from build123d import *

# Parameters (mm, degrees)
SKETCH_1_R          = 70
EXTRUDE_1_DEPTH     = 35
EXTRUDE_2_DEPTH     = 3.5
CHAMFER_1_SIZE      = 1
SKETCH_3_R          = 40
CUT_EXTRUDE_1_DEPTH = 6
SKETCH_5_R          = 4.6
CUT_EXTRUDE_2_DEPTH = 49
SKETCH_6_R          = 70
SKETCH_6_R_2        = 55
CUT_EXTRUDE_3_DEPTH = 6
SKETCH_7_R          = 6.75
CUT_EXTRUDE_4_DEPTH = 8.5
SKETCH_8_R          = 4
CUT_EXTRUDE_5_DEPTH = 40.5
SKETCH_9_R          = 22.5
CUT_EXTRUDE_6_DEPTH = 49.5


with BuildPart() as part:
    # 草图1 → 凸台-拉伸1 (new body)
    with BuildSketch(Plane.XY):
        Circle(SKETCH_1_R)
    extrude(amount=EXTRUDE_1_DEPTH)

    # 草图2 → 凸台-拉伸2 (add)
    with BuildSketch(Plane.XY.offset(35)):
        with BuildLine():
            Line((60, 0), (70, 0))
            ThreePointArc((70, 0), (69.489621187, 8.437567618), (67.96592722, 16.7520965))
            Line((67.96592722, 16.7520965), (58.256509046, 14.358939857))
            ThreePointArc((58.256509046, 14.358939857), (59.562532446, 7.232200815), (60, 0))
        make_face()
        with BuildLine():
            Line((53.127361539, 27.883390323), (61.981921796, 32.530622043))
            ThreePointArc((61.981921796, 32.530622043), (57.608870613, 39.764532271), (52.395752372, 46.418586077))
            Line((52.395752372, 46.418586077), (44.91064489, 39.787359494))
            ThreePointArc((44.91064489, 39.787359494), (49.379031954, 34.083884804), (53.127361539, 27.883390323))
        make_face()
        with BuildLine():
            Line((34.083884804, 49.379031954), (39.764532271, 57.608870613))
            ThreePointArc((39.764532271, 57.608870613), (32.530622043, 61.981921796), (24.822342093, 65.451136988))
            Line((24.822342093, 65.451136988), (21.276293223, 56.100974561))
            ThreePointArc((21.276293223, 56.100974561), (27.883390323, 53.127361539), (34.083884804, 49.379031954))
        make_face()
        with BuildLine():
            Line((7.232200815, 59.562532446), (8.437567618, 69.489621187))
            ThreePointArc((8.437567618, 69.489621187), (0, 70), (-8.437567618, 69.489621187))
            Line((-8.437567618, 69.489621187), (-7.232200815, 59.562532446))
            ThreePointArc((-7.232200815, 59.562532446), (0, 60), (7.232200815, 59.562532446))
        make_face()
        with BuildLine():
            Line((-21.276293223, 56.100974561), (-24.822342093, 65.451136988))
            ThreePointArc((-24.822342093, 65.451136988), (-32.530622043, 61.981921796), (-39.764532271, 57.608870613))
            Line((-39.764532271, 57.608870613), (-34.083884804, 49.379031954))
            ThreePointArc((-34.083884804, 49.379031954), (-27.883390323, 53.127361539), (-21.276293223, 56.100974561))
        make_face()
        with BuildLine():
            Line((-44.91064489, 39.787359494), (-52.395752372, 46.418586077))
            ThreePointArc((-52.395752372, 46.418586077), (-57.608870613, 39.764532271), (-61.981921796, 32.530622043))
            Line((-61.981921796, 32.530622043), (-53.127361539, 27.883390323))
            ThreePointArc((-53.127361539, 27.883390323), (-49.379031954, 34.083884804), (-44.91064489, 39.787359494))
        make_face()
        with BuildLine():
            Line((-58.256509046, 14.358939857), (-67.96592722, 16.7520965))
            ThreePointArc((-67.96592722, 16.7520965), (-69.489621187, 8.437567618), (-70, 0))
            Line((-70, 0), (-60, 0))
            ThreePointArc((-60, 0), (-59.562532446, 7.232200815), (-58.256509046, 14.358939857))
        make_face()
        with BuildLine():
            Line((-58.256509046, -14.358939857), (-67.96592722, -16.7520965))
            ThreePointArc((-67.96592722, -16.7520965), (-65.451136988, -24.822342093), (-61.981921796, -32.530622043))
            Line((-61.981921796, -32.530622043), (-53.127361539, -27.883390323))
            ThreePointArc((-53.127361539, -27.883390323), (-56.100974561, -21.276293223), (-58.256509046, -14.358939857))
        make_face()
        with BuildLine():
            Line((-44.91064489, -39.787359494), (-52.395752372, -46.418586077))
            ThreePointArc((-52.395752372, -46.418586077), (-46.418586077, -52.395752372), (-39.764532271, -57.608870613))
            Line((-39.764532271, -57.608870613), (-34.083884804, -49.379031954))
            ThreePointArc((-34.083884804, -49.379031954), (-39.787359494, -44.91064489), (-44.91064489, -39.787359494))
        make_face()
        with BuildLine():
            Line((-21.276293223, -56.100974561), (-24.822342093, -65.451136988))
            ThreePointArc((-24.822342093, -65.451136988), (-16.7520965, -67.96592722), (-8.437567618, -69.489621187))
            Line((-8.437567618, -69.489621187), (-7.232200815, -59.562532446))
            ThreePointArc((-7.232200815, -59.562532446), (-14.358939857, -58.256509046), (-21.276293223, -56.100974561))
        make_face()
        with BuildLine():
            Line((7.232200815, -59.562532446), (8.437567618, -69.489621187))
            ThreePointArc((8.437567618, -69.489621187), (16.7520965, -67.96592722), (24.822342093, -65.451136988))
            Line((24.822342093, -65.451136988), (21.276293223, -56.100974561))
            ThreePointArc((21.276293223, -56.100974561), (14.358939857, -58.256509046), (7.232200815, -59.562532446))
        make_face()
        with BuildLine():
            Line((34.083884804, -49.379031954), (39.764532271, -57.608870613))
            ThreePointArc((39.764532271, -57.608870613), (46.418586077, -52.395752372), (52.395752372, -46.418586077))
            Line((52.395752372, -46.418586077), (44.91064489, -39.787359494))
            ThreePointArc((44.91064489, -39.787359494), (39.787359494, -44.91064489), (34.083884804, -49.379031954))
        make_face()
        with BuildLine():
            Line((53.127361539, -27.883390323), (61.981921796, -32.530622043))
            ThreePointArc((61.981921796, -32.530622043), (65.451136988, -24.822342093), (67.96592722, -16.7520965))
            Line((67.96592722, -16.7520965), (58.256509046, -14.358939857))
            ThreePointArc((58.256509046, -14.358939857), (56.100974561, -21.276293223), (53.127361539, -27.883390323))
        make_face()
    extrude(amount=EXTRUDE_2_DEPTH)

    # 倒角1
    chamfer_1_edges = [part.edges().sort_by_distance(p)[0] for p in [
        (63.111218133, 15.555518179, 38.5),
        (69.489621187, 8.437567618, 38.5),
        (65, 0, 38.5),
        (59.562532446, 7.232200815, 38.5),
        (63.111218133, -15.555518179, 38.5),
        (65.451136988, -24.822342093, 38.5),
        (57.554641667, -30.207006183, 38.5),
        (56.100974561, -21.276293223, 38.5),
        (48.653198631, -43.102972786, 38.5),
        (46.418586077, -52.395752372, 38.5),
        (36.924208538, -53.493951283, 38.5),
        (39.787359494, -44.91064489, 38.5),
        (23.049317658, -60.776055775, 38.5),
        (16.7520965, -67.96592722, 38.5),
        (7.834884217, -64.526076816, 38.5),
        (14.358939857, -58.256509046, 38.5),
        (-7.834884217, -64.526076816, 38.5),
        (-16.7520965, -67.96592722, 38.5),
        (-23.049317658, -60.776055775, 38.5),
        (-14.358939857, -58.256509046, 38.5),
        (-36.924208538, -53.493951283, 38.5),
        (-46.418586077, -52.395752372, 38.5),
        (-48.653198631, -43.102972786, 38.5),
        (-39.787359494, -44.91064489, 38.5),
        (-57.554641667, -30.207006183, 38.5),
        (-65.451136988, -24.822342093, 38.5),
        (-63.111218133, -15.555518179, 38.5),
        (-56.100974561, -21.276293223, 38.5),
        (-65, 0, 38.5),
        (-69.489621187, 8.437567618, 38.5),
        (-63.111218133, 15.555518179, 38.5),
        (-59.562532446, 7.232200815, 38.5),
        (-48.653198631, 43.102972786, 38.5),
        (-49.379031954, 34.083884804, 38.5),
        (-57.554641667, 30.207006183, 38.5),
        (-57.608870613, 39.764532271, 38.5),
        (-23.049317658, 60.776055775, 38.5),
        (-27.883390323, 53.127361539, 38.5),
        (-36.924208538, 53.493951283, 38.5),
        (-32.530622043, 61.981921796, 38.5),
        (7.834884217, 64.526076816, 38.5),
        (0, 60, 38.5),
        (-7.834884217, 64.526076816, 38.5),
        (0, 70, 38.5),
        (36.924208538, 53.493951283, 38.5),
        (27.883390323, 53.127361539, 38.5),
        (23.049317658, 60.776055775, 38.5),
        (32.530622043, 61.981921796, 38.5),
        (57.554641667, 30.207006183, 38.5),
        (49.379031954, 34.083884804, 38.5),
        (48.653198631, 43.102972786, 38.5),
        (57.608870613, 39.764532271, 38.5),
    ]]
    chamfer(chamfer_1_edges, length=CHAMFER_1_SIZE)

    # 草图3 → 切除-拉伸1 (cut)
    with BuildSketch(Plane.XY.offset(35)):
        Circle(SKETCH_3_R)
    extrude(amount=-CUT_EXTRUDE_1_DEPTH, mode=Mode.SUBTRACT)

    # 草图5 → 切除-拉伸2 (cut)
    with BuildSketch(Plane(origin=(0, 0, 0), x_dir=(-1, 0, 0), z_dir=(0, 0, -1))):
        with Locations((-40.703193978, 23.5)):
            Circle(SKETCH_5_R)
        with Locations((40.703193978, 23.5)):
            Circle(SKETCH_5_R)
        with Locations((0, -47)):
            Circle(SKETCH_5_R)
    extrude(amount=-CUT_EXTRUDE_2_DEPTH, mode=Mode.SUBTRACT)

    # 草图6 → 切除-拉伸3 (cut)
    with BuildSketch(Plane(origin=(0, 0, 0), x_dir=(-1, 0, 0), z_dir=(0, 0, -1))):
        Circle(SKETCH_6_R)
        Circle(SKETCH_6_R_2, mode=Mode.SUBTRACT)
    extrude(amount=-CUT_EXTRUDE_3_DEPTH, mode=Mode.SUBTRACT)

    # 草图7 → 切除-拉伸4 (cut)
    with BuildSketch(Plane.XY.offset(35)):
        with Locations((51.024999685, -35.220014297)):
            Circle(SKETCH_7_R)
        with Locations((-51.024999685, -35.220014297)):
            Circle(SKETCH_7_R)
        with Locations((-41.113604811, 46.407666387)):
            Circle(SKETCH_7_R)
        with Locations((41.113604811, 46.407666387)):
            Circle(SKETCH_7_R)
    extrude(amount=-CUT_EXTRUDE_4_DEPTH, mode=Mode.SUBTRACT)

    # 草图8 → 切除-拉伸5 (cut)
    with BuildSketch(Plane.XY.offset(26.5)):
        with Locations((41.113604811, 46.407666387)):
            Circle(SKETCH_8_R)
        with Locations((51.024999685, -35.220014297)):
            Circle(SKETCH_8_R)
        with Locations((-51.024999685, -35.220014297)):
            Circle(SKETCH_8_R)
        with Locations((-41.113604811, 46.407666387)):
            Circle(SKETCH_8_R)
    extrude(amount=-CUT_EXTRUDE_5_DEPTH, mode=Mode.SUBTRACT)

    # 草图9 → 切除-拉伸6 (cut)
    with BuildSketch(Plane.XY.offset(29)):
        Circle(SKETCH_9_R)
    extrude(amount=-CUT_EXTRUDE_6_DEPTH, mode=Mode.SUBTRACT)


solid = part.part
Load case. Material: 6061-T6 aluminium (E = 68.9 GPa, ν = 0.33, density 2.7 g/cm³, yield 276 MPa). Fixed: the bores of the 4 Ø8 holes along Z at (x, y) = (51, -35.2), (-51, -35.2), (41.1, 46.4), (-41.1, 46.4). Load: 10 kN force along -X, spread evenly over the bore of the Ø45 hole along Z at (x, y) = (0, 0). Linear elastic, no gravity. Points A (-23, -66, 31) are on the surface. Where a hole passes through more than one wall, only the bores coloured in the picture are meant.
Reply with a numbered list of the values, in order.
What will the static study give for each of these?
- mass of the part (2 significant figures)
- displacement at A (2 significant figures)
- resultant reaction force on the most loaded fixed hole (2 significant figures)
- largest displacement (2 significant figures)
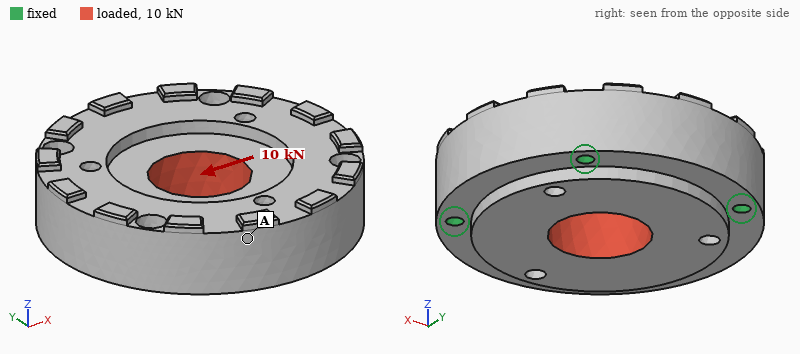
1. 1.1 kg
2. 0.83 µm
3. 2.8 kN
4. 3.1 µm
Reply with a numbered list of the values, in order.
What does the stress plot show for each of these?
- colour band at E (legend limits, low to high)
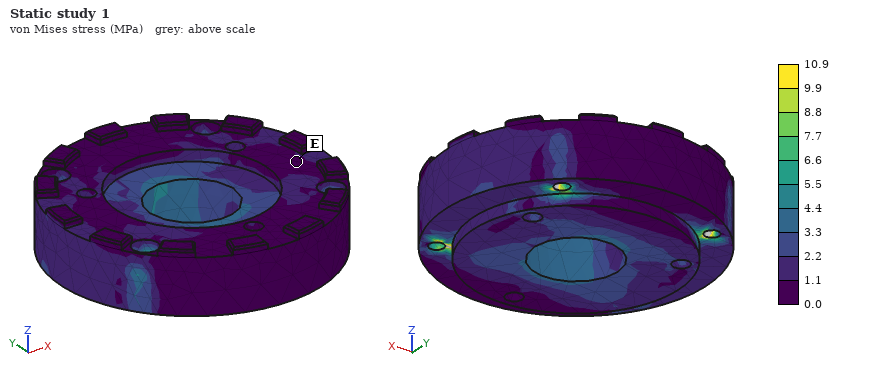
1. 0.0 to 1.1 MPa
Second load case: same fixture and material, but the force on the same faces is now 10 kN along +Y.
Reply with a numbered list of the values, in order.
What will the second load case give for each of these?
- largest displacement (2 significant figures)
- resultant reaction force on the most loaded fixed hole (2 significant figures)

1. 4.1 µm
2. 2.6 kN
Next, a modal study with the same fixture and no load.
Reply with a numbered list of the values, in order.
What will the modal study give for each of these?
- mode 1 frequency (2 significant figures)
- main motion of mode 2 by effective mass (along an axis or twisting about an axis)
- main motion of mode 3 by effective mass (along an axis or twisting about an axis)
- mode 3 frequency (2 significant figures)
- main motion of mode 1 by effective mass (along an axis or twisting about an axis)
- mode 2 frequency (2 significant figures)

1. 6600 Hz
2. along Z
3. twisting about X
4. 10 kHz
5. along Z
6. 8900 Hz
